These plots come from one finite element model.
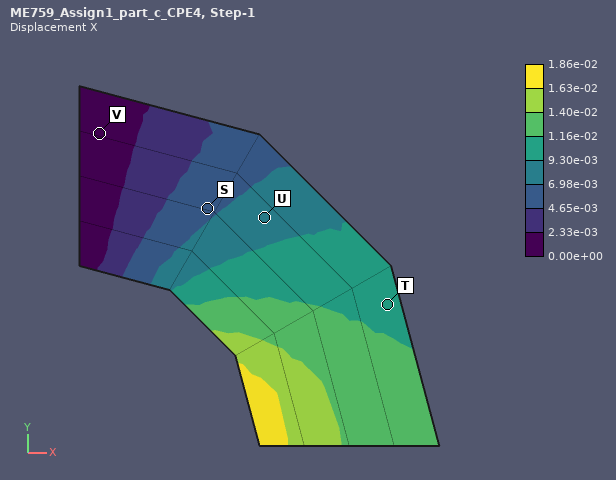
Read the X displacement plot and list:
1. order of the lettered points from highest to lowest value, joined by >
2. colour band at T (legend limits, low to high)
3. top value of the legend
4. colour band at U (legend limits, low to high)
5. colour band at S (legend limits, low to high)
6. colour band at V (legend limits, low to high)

T > U > S > V
9.30e-03 to 1.16e-02
1.86e-02
6.98e-03 to 9.30e-03
4.65e-03 to 6.98e-03
0.00e+00 to 2.33e-03
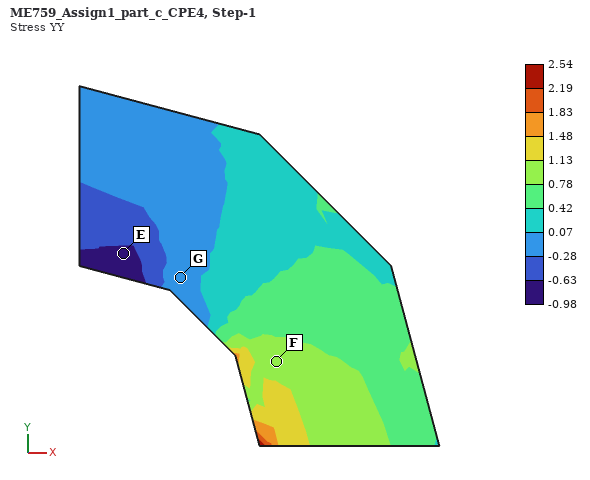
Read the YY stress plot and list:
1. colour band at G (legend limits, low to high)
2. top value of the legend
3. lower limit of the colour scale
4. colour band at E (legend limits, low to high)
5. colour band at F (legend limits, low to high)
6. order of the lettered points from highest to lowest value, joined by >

-0.28 to 0.07
2.54
-0.98
-0.98 to -0.63
0.78 to 1.13
F > G > E
